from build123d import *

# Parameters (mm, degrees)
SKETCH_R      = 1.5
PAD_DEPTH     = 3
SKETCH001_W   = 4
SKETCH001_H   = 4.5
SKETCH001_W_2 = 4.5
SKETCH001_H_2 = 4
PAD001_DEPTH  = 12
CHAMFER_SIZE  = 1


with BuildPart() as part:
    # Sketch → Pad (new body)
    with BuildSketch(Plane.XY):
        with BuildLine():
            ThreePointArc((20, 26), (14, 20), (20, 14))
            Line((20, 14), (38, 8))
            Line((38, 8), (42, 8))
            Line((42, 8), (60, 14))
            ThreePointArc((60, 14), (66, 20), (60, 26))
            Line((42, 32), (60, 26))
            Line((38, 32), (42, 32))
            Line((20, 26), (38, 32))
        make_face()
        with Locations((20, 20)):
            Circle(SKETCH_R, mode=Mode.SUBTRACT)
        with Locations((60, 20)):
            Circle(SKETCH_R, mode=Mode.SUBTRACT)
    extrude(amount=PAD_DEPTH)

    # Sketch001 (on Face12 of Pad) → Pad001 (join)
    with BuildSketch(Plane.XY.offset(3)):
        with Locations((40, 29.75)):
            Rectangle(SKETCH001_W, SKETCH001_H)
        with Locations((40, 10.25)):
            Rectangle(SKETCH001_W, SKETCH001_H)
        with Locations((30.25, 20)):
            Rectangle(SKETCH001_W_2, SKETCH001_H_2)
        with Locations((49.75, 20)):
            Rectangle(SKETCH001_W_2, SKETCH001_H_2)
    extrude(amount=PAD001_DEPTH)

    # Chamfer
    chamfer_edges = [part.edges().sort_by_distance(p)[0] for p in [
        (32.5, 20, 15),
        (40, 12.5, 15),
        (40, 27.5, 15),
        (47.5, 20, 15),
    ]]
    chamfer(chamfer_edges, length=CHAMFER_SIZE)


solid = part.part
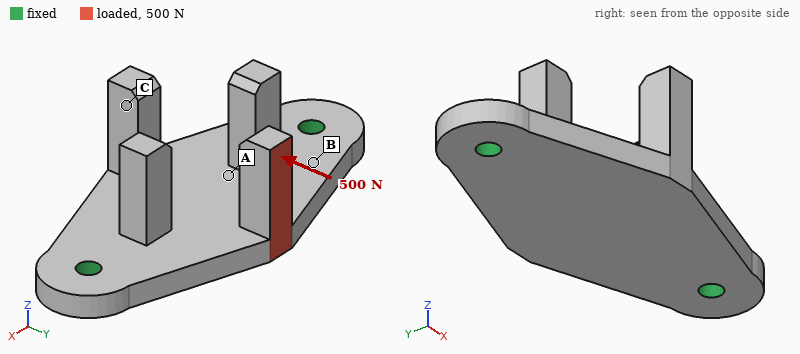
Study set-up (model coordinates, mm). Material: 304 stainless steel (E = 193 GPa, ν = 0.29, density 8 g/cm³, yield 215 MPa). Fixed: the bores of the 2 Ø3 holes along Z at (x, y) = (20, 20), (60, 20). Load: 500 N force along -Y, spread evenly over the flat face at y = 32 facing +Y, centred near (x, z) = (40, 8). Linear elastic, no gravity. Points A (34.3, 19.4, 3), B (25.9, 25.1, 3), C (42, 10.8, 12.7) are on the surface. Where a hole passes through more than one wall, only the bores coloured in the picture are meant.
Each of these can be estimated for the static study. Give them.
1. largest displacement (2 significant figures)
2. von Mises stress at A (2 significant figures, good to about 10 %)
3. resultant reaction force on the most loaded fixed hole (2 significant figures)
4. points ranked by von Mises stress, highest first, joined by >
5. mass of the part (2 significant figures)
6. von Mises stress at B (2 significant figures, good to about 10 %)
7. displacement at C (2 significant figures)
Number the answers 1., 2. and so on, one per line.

1. 97 µm
2. 38 MPa
3. 250 N
4. B > A > C
5. 27 g
6. 69 MPa
7. 23 µm
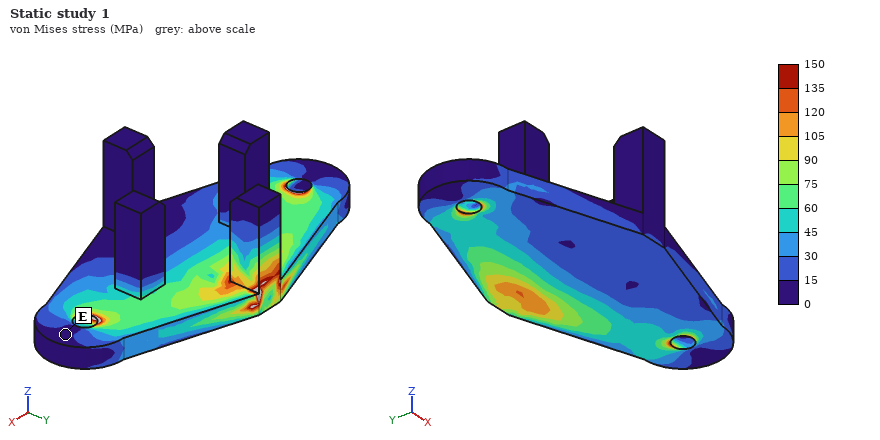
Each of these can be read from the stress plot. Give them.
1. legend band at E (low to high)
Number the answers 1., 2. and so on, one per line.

1. 0 to 15 MPa
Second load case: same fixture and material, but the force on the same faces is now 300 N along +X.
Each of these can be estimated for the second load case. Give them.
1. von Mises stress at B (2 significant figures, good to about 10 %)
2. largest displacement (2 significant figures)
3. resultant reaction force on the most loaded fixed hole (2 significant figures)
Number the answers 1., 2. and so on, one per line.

1. 12 MPa
2. 36 µm
3. 190 N
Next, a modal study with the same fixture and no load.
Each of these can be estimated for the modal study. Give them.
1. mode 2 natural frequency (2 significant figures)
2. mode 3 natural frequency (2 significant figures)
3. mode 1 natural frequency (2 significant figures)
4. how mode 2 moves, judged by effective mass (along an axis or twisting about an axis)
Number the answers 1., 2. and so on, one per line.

1. 6100 Hz
2. 11 kHz
3. 5500 Hz
4. along Z
